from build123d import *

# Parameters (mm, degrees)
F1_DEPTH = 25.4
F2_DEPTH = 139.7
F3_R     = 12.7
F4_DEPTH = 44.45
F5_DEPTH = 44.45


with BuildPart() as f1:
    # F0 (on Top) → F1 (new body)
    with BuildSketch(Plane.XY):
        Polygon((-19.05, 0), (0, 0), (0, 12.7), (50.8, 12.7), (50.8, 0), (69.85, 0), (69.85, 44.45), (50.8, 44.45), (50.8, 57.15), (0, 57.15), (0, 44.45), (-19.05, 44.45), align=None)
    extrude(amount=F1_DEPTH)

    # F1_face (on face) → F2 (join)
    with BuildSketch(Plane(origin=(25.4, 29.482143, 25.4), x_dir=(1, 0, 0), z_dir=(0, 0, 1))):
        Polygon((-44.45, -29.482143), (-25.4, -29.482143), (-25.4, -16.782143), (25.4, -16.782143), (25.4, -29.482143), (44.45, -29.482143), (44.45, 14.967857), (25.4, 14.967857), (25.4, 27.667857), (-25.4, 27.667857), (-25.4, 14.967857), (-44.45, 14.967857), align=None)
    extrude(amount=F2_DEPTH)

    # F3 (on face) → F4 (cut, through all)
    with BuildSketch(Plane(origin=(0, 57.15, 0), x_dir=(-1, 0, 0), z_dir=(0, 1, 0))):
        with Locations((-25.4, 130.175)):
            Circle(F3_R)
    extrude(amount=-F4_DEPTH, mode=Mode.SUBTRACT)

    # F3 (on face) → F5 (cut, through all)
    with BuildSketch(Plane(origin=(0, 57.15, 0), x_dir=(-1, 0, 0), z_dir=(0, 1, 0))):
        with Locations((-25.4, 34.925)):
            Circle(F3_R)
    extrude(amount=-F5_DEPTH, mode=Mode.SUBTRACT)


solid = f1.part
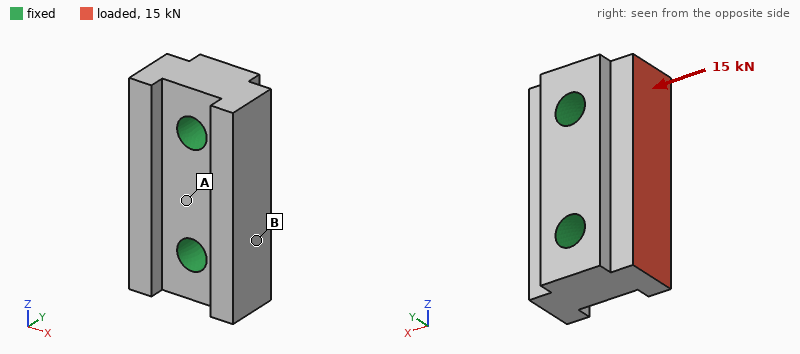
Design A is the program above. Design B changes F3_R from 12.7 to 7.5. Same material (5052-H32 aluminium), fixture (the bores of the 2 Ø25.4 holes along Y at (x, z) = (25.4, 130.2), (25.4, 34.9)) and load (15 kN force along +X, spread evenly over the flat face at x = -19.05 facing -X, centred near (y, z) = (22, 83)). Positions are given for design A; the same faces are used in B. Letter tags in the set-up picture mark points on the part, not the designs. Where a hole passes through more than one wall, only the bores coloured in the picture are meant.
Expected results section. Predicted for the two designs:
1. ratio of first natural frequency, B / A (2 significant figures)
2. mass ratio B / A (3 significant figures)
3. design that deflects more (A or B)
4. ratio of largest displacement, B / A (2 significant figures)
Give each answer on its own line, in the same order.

0.78
1.05
B
1.2
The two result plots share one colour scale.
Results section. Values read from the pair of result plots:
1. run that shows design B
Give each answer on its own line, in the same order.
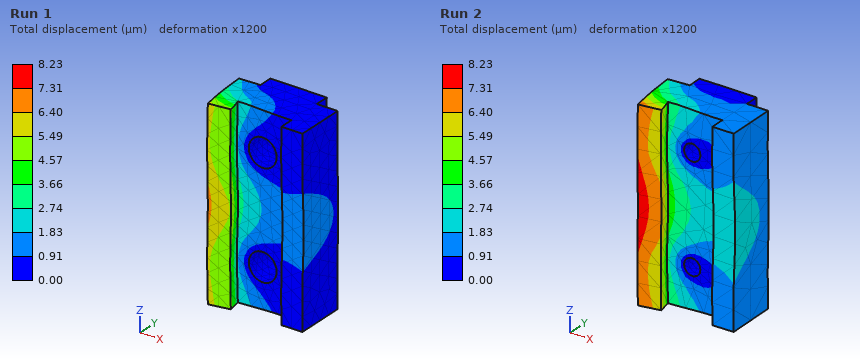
Run 2
